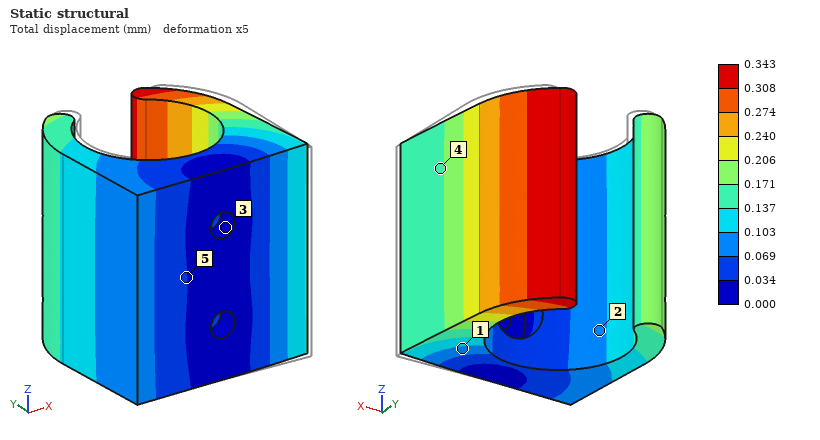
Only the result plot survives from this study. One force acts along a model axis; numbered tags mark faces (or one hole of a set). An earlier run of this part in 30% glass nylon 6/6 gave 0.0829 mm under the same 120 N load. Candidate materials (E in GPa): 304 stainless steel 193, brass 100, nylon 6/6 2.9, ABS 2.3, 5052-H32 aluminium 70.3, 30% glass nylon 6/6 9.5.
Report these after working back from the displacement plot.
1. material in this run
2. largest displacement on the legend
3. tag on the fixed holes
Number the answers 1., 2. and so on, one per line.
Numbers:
1. ABS
2. 0.343 mm
3. 3
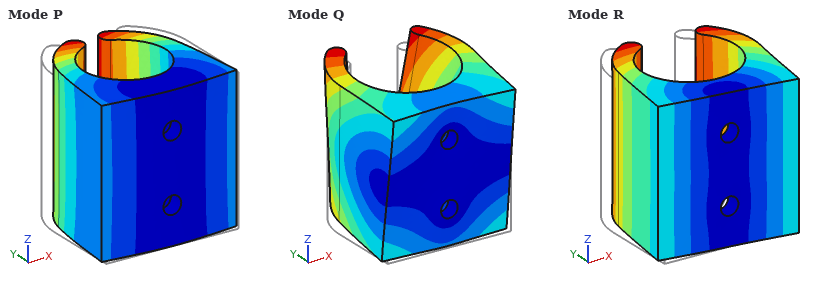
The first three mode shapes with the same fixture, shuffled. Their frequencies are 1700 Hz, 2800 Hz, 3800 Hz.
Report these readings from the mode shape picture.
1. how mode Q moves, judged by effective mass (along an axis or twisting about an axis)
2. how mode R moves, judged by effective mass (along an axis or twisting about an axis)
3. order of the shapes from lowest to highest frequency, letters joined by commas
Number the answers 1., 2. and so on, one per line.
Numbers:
1. along Z
2. along X
3. R, P, Q
